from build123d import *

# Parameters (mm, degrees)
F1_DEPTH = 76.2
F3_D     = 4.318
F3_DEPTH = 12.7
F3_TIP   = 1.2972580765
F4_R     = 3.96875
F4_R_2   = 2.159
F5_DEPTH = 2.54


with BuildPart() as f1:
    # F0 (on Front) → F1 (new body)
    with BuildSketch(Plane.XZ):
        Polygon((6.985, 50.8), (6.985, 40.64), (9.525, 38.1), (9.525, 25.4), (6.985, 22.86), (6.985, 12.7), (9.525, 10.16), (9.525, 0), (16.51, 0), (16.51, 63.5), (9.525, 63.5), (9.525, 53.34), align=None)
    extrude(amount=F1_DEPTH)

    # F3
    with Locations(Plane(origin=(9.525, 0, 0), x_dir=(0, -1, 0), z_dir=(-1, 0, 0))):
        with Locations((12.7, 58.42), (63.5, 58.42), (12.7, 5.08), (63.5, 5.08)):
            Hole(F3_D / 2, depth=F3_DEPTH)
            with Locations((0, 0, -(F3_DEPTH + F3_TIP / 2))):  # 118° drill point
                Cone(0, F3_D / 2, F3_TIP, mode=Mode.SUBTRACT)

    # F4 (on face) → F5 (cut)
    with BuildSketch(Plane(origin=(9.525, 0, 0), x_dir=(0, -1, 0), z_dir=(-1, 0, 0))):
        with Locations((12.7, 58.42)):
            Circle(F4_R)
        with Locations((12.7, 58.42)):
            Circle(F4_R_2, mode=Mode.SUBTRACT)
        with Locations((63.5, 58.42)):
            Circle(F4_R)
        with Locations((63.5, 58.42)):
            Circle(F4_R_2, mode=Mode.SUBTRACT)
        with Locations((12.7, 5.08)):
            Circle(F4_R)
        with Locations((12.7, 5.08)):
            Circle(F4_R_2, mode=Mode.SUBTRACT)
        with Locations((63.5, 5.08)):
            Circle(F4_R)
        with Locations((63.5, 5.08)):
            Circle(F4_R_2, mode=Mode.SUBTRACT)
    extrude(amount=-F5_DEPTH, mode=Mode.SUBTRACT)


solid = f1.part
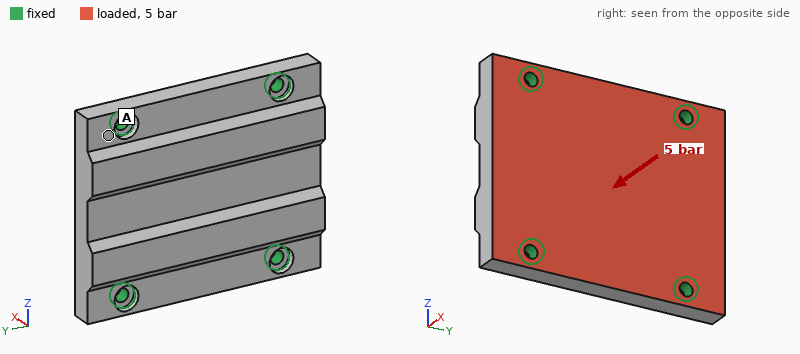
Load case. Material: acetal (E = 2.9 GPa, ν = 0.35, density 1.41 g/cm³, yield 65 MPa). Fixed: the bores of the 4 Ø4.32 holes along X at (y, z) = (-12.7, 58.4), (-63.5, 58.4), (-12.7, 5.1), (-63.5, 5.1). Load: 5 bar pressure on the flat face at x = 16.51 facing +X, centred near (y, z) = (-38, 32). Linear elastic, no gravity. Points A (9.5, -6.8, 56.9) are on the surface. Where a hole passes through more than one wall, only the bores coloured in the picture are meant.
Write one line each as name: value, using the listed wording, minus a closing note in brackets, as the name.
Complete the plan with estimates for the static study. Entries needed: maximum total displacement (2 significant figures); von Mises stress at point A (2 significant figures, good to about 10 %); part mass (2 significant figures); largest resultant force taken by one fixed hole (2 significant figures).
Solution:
maximum total displacement: 0.36 mm
von Mises stress at point A: 5.8 MPa
part mass: 54 g
largest resultant force taken by one fixed hole: 680 N
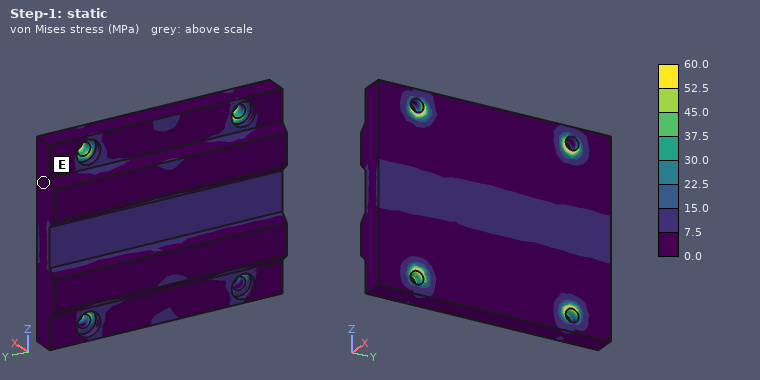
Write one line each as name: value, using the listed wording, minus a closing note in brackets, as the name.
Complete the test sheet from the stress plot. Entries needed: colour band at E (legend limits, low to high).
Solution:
colour band at E: 0.0 to 7.5 MPa
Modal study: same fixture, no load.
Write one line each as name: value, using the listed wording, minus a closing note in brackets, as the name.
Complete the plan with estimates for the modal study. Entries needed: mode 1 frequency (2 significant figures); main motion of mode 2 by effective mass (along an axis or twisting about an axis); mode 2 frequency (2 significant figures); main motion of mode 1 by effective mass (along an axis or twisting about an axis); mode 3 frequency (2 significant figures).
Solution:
mode 1 frequency: 2100 Hz
main motion of mode 2 by effective mass: twisting about Z
mode 2 frequency: 2800 Hz
main motion of mode 1 by effective mass: along X
mode 3 frequency: 3000 Hz
